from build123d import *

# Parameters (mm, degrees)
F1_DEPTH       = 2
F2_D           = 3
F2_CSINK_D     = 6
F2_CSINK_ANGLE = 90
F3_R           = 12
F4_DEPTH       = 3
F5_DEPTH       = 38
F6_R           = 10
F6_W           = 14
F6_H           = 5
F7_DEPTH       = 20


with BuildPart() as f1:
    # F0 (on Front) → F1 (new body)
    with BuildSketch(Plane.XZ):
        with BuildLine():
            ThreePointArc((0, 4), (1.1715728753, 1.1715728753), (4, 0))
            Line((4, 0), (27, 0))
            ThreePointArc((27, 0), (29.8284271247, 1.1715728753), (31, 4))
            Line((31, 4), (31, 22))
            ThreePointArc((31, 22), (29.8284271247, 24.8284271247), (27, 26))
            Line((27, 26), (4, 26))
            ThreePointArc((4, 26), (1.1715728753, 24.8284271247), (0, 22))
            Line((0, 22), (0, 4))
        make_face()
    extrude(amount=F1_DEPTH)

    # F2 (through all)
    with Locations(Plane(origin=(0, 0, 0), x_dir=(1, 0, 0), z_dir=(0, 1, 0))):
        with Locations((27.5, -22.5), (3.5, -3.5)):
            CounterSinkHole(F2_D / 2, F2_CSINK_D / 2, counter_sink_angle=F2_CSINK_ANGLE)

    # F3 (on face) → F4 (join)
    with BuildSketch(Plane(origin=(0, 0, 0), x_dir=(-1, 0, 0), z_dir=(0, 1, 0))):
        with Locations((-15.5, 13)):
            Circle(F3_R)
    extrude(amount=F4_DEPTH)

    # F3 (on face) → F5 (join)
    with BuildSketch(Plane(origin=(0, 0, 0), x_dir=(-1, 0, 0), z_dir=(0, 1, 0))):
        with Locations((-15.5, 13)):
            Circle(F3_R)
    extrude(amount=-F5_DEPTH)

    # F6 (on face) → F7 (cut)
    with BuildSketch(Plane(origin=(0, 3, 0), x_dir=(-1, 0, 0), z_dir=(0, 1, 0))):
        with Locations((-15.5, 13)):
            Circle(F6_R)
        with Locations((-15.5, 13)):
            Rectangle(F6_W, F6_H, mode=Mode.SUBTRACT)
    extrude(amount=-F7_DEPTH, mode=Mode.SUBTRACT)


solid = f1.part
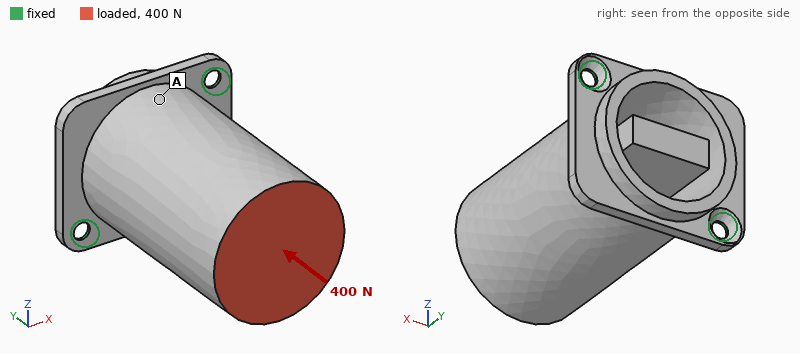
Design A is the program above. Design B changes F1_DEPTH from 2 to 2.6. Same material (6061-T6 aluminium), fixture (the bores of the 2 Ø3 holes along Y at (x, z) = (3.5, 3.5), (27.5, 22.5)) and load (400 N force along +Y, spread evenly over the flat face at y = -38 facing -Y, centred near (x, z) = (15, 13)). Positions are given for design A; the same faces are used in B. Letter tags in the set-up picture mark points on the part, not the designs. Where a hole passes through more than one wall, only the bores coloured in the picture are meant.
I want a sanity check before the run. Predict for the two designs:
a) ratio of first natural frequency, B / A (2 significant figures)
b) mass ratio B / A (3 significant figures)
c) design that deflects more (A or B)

1.6
1.01
A
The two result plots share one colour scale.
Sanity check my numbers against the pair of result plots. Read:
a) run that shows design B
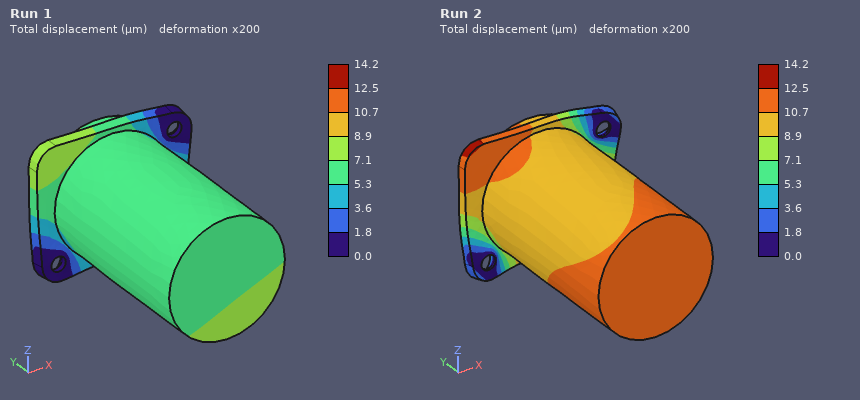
Run 1
